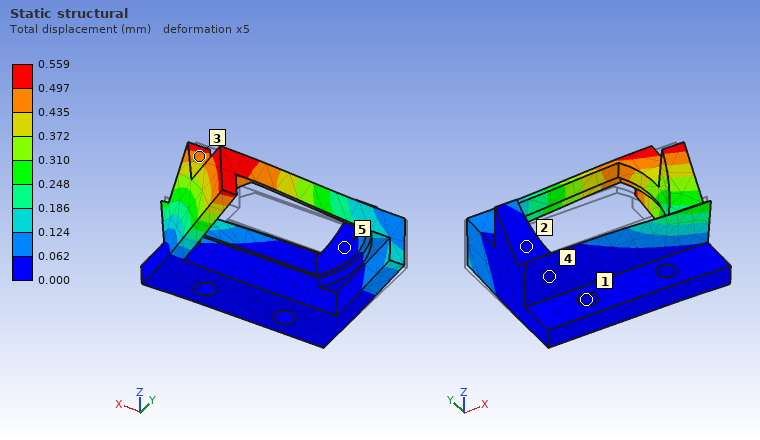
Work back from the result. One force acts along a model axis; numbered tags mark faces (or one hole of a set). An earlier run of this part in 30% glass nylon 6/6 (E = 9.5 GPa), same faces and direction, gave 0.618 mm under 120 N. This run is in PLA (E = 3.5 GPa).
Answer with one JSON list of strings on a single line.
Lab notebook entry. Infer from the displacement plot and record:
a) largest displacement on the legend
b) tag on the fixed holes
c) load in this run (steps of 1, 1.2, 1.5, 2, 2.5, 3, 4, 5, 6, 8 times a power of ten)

["0.559 mm", "1", "40 N"]
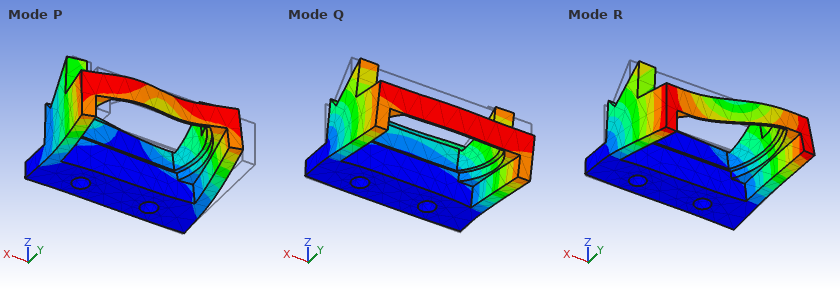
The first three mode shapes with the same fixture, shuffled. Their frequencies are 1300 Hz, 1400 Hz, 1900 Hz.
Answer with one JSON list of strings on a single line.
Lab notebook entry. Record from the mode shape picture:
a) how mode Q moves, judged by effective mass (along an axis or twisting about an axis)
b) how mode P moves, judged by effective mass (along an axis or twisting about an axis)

["along Z", "along X"]
